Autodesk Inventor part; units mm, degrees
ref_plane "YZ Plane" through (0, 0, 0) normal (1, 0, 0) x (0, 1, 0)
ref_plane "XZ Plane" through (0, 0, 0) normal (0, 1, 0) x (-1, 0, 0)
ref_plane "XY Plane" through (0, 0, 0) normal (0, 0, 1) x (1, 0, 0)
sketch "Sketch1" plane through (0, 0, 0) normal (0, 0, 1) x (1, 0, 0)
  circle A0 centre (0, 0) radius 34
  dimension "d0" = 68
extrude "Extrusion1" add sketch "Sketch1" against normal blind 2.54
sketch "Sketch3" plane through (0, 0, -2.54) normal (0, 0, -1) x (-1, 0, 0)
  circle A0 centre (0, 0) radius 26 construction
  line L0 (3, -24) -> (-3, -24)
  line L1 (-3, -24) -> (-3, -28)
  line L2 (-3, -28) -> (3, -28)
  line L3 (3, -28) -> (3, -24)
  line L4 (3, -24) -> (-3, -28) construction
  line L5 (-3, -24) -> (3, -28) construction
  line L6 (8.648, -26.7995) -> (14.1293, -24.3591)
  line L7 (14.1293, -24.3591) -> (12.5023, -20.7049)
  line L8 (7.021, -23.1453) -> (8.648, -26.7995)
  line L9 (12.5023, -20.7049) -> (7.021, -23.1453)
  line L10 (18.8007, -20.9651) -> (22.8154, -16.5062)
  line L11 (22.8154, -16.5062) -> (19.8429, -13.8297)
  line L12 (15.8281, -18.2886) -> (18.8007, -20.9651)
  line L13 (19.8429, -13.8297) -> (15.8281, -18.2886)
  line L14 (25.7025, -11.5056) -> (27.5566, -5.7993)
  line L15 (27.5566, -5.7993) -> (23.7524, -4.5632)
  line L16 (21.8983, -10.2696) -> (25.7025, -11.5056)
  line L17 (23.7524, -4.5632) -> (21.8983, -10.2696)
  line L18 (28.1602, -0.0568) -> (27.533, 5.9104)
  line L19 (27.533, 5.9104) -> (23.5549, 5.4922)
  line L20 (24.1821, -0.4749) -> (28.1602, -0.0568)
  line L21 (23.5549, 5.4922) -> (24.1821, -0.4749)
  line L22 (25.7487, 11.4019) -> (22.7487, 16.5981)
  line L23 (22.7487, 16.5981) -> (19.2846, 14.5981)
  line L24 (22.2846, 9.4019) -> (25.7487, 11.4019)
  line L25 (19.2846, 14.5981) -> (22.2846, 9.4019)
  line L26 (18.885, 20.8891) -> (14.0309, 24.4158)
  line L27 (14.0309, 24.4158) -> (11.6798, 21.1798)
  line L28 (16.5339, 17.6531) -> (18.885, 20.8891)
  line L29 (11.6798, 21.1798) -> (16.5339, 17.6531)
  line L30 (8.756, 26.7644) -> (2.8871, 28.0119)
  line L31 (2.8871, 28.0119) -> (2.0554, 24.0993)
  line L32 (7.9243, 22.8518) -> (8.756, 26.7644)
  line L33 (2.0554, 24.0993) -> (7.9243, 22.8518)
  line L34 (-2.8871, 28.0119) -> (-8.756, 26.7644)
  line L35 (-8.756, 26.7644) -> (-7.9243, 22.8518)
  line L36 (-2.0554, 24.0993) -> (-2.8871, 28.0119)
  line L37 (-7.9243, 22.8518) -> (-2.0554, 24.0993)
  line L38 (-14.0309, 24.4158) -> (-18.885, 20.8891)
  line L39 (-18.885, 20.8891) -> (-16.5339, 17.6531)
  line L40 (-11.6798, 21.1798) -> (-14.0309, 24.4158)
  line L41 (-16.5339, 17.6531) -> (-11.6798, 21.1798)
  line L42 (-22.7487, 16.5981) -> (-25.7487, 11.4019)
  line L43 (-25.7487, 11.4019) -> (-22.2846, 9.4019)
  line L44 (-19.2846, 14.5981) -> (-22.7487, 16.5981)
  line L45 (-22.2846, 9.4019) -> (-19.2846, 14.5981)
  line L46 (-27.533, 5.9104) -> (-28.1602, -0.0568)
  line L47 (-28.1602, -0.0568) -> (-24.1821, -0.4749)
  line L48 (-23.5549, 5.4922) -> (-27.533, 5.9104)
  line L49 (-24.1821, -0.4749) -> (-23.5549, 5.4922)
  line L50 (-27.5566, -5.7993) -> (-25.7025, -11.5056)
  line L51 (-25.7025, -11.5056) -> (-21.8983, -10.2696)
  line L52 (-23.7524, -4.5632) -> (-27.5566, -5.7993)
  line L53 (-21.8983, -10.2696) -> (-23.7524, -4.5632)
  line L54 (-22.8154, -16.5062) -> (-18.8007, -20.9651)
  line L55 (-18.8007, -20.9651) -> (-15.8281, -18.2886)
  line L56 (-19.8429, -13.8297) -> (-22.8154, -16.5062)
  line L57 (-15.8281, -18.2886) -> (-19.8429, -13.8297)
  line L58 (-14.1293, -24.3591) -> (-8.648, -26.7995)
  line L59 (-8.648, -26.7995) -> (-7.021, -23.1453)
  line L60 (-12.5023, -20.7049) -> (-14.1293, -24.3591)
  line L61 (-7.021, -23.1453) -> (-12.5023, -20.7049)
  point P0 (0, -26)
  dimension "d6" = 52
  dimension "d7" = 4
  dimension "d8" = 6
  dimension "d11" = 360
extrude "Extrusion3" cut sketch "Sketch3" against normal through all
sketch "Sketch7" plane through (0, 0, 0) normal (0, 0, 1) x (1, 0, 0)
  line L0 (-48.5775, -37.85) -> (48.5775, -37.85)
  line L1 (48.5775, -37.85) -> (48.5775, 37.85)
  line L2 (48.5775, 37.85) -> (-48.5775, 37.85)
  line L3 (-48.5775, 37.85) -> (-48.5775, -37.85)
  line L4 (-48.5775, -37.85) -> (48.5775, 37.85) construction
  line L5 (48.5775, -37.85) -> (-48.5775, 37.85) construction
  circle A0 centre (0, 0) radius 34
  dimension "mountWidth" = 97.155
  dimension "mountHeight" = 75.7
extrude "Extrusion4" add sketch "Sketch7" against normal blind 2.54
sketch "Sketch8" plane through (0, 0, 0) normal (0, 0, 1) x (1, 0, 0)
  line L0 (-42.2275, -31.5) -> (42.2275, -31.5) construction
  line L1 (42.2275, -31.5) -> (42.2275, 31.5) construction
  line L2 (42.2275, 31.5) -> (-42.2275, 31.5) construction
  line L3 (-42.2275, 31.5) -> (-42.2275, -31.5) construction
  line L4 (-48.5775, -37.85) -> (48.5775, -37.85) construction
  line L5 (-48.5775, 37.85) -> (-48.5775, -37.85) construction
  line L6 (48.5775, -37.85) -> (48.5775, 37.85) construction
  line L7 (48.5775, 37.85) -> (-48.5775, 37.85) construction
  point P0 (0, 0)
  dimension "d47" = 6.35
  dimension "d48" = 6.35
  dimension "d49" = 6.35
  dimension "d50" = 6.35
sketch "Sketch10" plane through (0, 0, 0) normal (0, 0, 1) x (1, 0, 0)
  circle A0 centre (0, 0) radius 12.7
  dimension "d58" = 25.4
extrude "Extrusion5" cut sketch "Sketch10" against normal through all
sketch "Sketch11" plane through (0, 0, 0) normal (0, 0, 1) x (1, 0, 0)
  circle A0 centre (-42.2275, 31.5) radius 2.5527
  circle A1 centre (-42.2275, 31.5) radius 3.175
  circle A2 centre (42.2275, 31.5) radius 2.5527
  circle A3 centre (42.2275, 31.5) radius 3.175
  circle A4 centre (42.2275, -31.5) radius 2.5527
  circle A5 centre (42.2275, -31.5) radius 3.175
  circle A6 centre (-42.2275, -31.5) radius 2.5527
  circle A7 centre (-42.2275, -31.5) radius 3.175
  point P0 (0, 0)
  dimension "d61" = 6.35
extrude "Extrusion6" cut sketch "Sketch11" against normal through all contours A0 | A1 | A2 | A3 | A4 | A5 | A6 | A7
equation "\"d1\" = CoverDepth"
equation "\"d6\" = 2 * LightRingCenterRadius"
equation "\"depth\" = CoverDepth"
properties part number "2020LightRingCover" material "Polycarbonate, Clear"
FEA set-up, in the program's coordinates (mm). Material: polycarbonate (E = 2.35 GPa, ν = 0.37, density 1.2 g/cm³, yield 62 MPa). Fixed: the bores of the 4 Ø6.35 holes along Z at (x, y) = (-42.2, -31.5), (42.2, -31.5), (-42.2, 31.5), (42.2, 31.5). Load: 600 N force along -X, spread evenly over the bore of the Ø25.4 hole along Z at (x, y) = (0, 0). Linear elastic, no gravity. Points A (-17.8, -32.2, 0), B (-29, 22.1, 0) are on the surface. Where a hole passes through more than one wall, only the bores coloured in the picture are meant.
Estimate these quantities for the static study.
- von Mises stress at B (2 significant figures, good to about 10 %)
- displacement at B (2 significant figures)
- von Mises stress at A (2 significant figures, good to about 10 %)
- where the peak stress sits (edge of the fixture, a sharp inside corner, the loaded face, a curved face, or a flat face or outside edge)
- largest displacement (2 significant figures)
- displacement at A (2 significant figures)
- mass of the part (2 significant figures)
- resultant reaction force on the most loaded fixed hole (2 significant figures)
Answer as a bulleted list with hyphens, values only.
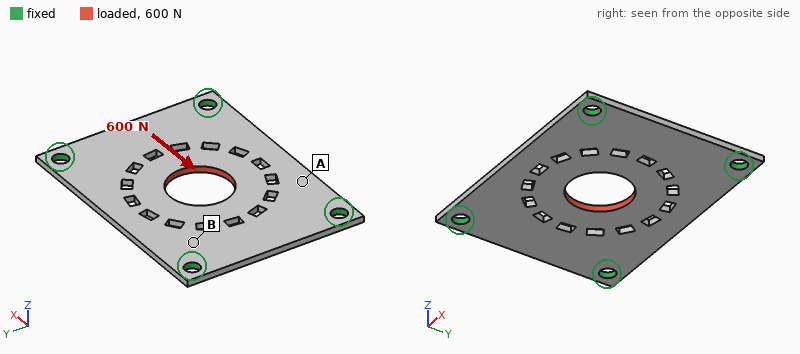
- 3.1 MPa
- 27 µm
- 1.4 MPa
- edge of the fixture
- 76 µm
- 23 µm
- 19 g
- 160 N
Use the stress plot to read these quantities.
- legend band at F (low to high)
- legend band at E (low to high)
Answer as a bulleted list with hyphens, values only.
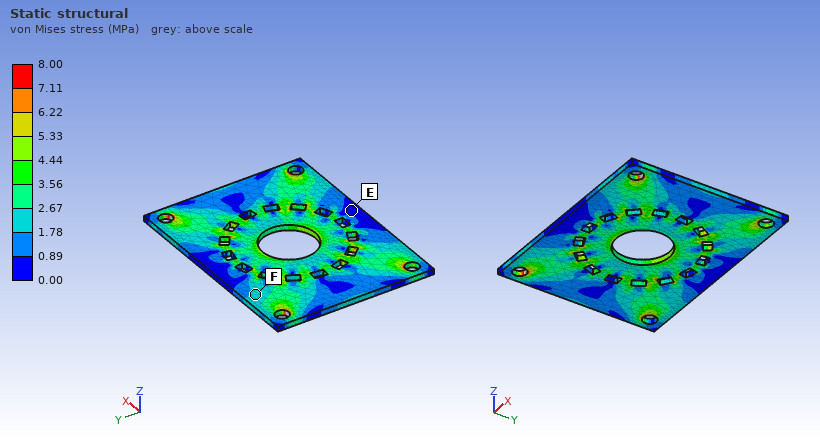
- 1.78 to 2.67 MPa
- 0.00 to 0.89 MPa
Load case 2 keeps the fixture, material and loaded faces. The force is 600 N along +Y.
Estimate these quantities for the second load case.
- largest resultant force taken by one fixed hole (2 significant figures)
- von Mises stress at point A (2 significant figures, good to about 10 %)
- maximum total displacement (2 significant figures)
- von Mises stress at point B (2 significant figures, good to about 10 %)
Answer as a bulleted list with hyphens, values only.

- 180 N
- 1.8 MPa
- 0.12 mm
- 3.4 MPa
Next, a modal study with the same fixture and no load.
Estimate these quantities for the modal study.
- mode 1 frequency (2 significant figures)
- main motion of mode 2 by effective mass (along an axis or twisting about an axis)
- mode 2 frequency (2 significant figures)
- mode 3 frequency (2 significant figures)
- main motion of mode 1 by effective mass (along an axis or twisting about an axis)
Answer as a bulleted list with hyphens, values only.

- 470 Hz
- twisting about X
- 660 Hz
- 910 Hz
- along Z
